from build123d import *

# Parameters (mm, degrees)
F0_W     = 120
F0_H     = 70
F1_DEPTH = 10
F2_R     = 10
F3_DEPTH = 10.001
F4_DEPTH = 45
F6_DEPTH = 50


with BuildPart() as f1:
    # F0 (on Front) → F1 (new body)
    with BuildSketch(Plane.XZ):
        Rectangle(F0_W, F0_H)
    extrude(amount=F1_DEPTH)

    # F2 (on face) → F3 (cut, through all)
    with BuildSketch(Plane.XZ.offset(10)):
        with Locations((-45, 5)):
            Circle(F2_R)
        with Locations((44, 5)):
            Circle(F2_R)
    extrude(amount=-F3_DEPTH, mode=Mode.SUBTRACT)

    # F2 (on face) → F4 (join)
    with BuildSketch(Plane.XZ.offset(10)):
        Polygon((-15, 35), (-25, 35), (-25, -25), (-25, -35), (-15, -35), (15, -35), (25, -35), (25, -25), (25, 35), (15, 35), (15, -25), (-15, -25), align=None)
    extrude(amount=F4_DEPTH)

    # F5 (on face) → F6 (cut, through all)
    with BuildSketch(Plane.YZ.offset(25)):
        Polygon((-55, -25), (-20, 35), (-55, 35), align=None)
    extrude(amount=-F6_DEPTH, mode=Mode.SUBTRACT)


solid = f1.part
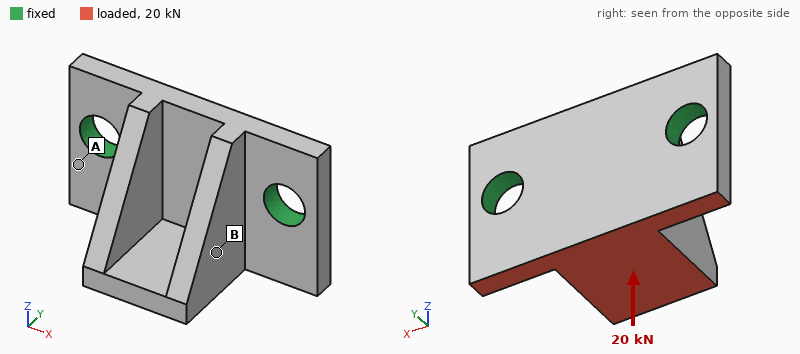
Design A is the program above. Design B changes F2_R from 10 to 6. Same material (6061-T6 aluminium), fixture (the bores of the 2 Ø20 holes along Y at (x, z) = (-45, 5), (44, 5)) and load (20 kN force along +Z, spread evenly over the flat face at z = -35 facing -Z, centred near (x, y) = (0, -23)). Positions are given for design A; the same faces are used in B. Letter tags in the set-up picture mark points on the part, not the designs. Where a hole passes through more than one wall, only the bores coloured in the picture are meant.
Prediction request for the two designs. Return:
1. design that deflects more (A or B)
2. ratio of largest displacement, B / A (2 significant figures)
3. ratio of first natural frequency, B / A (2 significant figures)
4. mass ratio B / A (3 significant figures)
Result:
B
1.5
0.78
1.03
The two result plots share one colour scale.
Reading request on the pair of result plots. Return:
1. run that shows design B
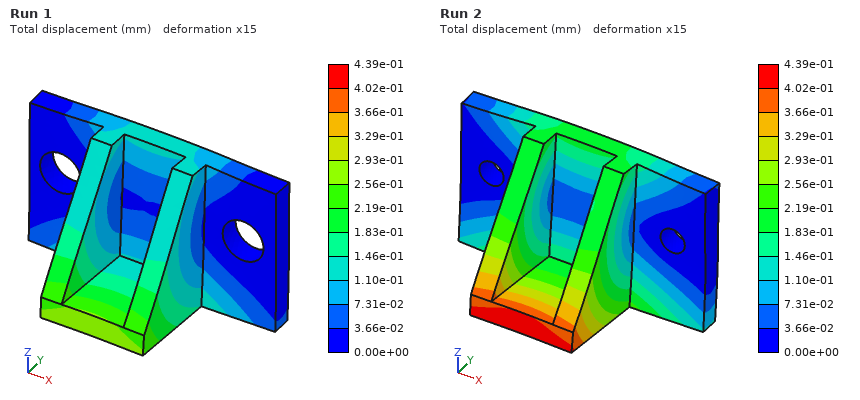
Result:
Run 2
